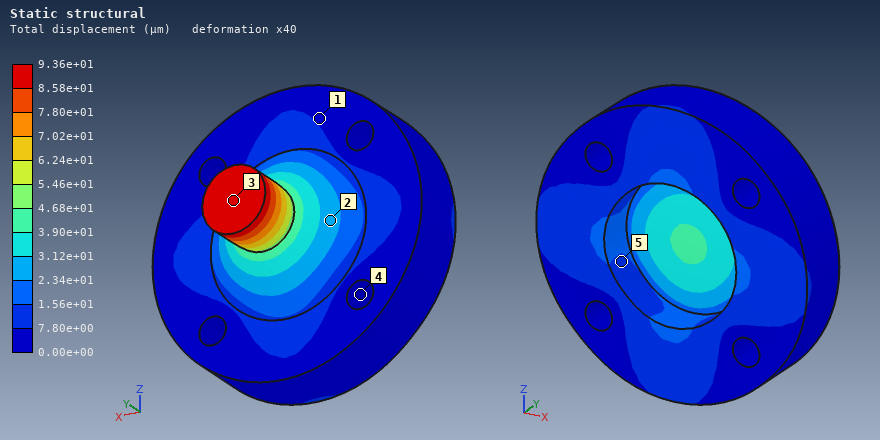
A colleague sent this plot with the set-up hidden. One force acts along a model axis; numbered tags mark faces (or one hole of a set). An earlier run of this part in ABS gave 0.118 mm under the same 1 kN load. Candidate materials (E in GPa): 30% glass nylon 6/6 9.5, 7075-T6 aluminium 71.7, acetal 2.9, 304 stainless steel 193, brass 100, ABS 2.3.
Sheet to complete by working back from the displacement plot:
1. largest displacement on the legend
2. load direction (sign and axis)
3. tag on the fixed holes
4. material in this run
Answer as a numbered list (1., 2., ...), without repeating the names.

1. 9.36e+01 µm
2. -Y
3. 4
4. acetal
